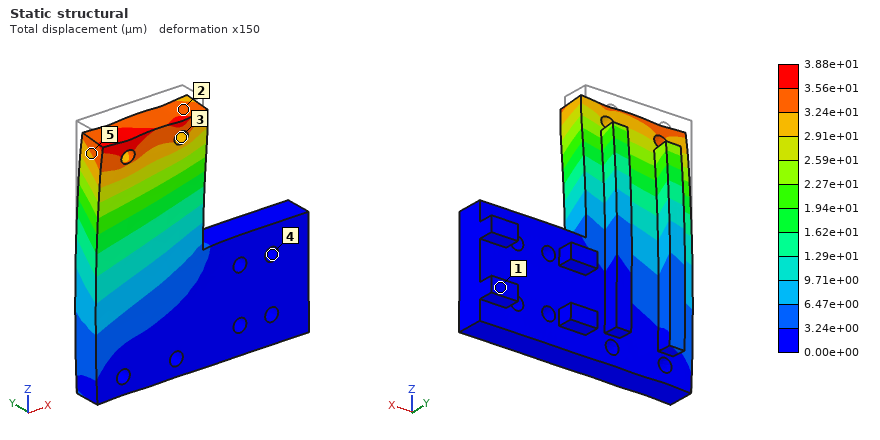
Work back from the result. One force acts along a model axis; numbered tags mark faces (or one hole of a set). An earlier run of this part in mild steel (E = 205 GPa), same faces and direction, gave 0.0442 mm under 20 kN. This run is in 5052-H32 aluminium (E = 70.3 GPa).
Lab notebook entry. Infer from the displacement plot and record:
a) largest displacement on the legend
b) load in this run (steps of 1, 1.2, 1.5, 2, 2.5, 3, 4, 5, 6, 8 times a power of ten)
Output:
3.88e+01 µm
6 kN
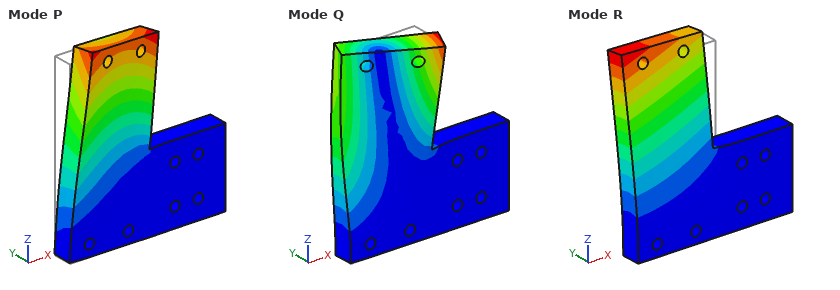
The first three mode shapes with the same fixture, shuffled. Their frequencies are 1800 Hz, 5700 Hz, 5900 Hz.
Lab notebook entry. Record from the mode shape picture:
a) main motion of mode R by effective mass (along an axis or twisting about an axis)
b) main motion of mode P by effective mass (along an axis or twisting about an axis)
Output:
along Y
along X
